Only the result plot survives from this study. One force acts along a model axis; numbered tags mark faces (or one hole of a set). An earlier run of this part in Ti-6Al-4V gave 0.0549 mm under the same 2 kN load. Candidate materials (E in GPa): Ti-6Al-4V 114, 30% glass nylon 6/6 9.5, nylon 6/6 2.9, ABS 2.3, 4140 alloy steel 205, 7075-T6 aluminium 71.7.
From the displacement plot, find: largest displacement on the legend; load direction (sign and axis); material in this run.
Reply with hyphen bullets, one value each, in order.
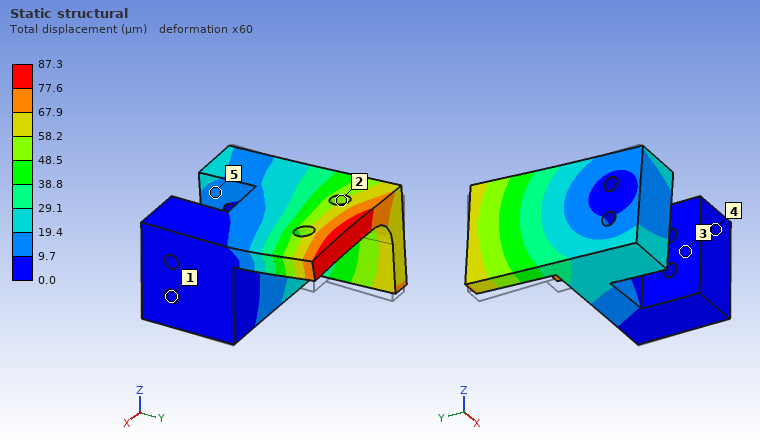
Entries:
- 87.3 µm
- +Z
- 7075-T6 aluminium
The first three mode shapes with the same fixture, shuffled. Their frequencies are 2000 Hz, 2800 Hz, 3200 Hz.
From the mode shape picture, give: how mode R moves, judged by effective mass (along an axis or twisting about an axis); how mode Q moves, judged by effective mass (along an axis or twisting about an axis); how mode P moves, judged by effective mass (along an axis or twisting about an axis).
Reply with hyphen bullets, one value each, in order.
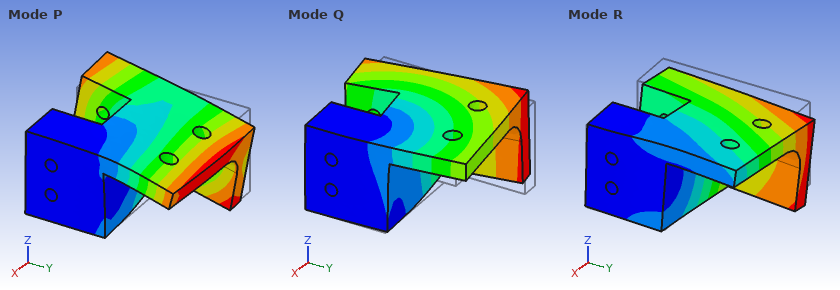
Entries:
- along Z
- along Y
- twisting about X
